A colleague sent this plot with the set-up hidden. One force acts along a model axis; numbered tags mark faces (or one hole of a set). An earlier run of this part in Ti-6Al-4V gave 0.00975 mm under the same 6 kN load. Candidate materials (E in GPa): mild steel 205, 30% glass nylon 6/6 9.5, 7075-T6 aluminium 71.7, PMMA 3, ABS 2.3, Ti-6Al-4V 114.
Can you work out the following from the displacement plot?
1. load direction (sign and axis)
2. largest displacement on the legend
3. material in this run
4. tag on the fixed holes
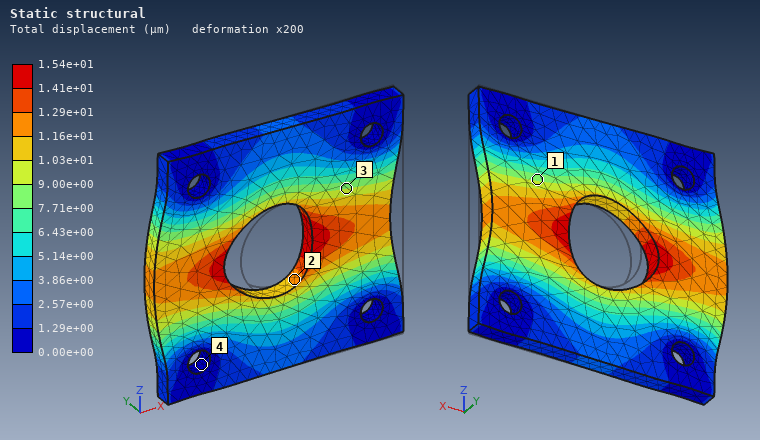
-X
1.54e+01 µm
7075-T6 aluminium
4
